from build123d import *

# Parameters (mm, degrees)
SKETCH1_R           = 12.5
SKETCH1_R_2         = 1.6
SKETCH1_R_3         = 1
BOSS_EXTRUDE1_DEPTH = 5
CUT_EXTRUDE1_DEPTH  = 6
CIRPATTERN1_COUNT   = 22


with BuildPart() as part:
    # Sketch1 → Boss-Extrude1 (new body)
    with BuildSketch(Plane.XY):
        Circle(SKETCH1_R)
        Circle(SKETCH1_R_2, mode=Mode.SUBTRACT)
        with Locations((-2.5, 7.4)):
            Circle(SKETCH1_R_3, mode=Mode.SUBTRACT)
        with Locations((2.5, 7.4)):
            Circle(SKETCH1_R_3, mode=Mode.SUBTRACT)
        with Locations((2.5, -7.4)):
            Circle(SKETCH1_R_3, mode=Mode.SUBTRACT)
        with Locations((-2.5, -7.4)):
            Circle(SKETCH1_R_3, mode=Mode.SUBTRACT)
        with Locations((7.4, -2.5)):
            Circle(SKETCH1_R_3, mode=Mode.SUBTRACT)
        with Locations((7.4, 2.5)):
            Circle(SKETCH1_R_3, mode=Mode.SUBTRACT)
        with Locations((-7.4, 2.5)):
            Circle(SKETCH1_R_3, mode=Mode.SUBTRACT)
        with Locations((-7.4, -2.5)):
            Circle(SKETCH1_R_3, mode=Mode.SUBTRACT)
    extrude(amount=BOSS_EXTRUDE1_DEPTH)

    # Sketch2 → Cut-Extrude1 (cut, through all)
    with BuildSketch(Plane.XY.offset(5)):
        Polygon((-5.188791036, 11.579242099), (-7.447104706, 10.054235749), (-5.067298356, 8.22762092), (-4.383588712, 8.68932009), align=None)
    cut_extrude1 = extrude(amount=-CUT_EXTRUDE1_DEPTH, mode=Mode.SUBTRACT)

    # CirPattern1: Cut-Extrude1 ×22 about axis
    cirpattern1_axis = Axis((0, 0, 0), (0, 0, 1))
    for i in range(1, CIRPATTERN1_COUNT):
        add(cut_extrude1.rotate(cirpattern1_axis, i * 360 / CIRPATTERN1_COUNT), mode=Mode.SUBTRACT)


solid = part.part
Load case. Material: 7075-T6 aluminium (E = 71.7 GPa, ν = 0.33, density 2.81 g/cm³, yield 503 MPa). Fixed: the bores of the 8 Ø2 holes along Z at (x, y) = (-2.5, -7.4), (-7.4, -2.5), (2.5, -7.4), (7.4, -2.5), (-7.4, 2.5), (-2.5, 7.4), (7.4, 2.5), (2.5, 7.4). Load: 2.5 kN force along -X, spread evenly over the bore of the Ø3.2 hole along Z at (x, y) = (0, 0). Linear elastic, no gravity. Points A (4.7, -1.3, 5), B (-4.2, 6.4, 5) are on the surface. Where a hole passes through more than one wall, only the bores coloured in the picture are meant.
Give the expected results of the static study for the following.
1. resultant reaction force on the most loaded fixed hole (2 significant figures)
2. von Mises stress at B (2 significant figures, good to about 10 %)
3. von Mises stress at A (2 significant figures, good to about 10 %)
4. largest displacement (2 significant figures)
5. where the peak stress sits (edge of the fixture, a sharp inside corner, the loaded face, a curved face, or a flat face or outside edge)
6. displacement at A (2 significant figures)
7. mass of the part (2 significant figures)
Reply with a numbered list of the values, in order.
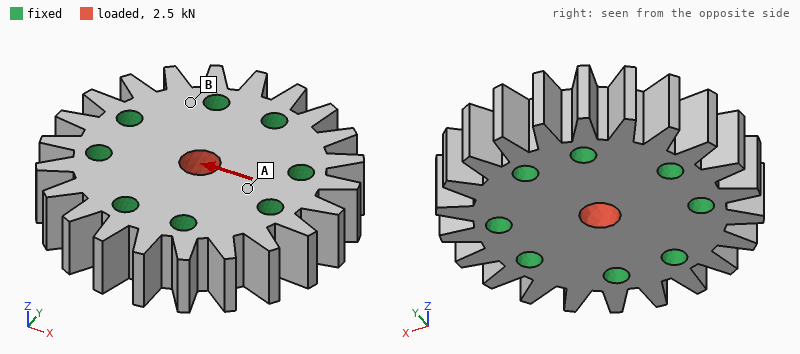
1. 520 N
2. 9.6 MPa
3. 30 MPa
4. 2.8 µm
5. the loaded face
6. 0.95 µm
7. 4.9 g
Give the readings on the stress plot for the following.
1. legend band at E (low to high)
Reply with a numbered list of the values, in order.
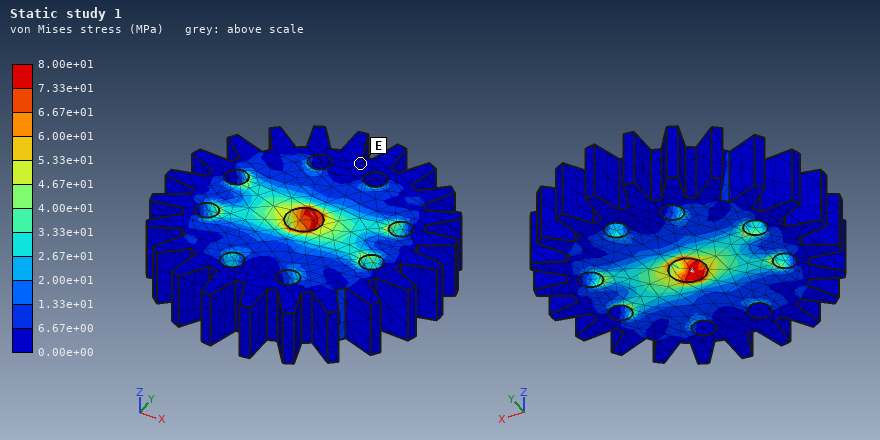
1. 0.00e+00 to 6.67e+00 MPa
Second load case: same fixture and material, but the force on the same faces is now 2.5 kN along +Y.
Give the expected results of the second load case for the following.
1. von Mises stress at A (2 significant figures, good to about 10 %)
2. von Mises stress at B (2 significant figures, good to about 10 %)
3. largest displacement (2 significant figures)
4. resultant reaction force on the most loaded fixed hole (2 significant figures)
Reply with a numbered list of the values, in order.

1. 11 MPa
2. 11 MPa
3. 2.8 µm
4. 520 N
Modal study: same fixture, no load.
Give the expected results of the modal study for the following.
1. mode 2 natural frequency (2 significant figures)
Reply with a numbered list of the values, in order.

1. 120 kHz
